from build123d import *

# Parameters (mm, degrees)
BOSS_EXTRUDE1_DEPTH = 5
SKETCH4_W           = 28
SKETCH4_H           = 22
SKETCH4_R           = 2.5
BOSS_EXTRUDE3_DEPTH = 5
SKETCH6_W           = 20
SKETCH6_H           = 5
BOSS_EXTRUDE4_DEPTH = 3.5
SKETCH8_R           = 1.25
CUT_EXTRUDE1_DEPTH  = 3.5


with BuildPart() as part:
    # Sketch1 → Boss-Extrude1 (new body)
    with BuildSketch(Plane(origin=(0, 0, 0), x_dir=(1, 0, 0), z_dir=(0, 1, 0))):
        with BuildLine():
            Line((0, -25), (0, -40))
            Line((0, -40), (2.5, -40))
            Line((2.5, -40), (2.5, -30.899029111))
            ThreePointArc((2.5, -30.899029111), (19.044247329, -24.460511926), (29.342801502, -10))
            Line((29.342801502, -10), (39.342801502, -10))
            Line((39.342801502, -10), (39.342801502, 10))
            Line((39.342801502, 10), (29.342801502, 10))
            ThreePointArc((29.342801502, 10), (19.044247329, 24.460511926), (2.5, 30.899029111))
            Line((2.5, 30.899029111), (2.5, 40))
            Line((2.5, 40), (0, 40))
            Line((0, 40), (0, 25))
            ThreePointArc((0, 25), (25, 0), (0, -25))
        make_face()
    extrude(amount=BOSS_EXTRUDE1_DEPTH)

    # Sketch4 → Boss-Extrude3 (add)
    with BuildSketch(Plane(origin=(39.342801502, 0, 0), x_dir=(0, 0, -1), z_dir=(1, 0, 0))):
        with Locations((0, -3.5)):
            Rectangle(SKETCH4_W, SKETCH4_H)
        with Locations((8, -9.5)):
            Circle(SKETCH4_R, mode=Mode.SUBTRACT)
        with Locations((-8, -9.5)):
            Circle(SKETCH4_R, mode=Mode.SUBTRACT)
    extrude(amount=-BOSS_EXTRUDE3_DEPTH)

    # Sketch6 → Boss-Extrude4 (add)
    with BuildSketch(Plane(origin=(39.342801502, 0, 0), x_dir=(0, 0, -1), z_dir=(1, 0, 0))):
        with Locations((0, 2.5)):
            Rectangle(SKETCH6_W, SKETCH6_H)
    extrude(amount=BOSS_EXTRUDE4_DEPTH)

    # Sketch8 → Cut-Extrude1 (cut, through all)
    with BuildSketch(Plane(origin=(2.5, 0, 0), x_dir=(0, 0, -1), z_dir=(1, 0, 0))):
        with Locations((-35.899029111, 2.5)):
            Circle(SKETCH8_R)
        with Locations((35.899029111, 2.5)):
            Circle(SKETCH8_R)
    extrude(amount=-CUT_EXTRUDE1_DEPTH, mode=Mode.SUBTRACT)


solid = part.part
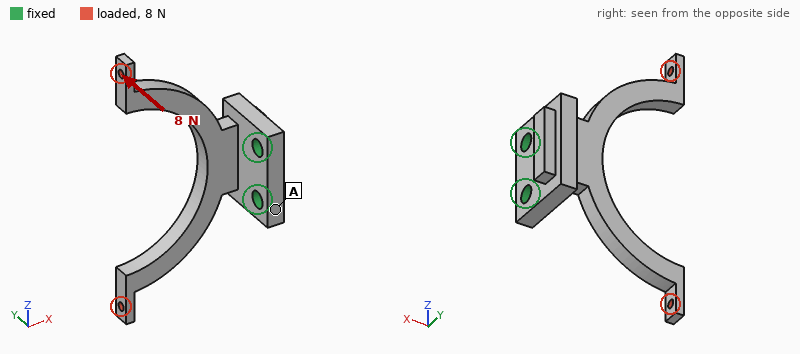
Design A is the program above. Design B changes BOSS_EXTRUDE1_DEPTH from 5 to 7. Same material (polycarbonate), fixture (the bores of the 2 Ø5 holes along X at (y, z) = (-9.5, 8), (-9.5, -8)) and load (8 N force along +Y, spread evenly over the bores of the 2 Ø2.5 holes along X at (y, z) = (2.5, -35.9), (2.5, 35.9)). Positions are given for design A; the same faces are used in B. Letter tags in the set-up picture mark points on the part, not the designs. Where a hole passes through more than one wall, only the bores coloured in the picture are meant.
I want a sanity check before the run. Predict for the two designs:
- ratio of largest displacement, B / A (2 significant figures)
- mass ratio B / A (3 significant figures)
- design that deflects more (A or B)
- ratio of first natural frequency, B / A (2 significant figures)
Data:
0.47
1.20
A
1.1
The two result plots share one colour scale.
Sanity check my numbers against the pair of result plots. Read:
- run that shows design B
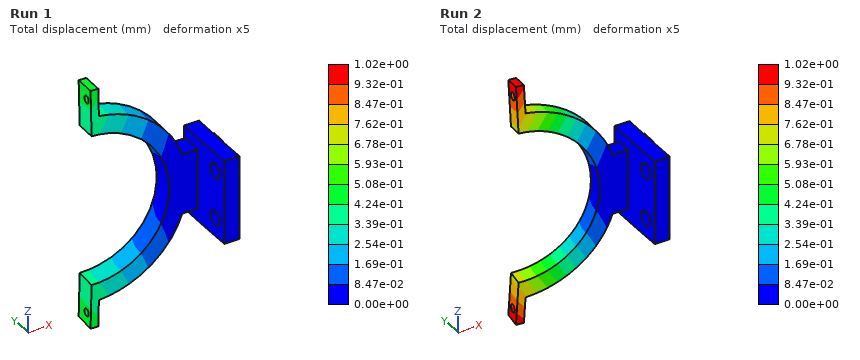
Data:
Run 1
